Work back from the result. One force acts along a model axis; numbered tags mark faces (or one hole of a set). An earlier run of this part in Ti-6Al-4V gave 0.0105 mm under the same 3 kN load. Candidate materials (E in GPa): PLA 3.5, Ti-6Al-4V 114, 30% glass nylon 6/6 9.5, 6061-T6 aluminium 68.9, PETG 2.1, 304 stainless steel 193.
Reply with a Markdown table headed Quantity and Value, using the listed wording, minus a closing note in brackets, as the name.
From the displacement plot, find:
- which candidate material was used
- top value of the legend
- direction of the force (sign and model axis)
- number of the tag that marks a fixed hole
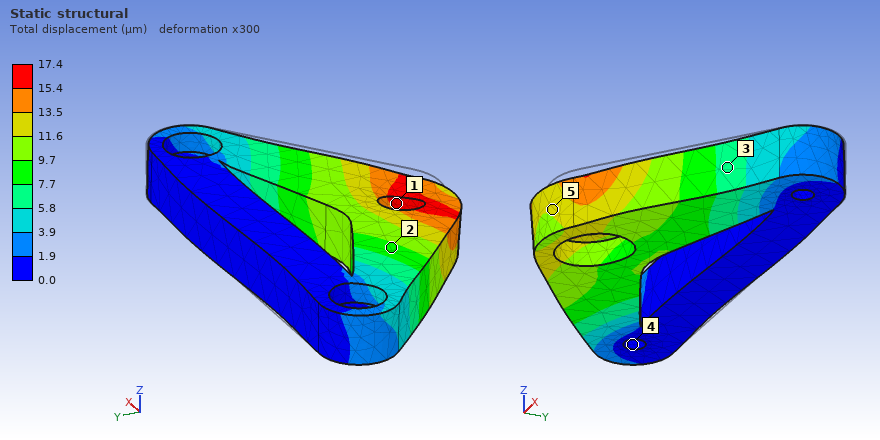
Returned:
| Quantity | Value |
|---|---|
| which candidate material was used | 6061-T6 aluminium |
| top value of the legend | 17.4 µm |
| direction of the force | -X |
| number of the tag that marks a fixed hole | 4 |
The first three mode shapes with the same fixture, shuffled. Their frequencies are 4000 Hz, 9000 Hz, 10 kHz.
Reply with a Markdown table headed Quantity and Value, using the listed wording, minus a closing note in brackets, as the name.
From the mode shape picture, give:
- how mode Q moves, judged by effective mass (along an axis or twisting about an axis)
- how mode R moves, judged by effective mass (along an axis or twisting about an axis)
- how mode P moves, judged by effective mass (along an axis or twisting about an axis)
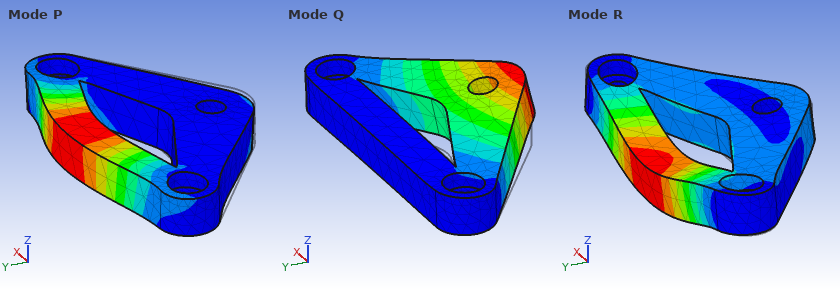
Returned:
| Quantity | Value |
|---|---|
| how mode Q moves, judged by effective mass | along Z |
| how mode R moves, judged by effective mass | along Z |
| how mode P moves, judged by effective mass | along Y |
